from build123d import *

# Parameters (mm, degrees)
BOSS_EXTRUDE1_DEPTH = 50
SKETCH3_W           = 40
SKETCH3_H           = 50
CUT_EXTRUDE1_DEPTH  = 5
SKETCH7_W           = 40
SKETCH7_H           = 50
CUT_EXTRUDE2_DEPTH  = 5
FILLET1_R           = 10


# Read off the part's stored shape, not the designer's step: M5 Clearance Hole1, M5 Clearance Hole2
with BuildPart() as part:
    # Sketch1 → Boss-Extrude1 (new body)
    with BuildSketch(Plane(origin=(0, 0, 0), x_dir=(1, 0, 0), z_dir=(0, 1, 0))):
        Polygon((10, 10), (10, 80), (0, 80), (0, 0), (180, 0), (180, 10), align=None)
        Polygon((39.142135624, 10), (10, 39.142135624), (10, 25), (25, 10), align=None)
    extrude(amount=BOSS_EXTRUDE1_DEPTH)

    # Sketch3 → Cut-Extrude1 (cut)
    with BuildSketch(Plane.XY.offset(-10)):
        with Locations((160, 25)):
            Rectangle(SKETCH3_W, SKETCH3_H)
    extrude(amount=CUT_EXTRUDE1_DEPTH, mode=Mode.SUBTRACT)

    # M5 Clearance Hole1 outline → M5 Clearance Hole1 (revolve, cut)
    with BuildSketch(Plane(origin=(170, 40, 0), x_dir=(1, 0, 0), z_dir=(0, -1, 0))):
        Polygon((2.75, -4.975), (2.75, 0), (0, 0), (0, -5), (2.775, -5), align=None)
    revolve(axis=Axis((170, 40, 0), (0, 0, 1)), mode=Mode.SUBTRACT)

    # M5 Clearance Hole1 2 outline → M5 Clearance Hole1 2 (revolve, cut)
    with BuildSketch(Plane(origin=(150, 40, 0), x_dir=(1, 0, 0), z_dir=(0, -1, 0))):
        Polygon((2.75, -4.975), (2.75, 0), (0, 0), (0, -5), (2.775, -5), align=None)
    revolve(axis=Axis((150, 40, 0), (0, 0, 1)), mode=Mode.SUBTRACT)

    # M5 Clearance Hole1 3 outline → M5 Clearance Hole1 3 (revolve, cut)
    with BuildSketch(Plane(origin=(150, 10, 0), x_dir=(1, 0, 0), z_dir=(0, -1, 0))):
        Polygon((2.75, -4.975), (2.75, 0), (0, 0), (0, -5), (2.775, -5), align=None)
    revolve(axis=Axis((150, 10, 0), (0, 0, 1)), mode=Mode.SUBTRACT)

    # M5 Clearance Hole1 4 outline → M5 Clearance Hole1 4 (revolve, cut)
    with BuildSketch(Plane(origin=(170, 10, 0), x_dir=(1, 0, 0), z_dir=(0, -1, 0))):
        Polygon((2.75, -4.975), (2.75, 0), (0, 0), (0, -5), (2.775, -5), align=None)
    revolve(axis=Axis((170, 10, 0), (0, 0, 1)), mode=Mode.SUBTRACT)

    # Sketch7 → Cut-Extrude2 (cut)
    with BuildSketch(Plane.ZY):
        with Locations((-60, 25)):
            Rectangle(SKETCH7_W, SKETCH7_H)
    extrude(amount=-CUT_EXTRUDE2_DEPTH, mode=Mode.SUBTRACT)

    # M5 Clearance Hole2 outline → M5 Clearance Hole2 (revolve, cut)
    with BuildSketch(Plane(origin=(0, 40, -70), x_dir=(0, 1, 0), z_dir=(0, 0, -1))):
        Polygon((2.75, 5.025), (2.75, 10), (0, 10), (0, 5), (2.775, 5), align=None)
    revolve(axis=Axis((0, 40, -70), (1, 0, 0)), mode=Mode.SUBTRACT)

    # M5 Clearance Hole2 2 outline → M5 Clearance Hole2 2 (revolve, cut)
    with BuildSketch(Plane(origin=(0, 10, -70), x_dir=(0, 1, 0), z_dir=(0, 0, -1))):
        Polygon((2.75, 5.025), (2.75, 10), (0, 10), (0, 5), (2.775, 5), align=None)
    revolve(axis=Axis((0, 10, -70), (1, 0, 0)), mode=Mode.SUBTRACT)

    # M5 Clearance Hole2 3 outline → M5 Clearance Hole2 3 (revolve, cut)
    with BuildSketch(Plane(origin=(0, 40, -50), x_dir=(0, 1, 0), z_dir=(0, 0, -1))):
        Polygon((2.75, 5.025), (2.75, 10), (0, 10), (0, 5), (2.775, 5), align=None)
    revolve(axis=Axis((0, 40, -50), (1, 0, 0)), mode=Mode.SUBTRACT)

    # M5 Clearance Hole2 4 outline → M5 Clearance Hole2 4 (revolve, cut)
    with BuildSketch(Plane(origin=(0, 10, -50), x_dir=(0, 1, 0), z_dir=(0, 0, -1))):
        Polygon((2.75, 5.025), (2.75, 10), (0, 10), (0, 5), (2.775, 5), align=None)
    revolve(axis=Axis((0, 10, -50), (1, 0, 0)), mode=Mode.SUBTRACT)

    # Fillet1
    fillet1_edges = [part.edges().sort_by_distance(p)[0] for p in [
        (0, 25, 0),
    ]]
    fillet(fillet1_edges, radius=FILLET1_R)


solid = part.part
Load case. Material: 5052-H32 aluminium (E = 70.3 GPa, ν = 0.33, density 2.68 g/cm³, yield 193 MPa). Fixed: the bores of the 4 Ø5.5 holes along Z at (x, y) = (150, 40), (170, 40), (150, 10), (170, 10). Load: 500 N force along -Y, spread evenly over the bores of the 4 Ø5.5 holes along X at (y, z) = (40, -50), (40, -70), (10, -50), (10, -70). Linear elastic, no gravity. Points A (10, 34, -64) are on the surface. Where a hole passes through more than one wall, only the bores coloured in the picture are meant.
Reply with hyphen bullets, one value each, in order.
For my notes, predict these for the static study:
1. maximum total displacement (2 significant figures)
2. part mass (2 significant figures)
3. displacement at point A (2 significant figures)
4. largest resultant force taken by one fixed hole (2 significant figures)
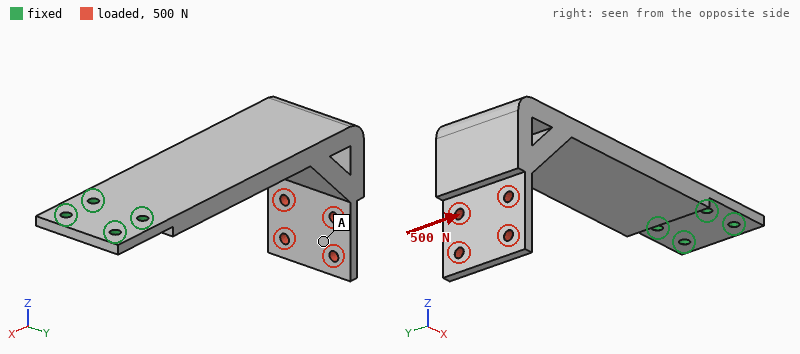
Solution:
- 0.69 mm
- 320 g
- 0.54 mm
- 2.1 kN
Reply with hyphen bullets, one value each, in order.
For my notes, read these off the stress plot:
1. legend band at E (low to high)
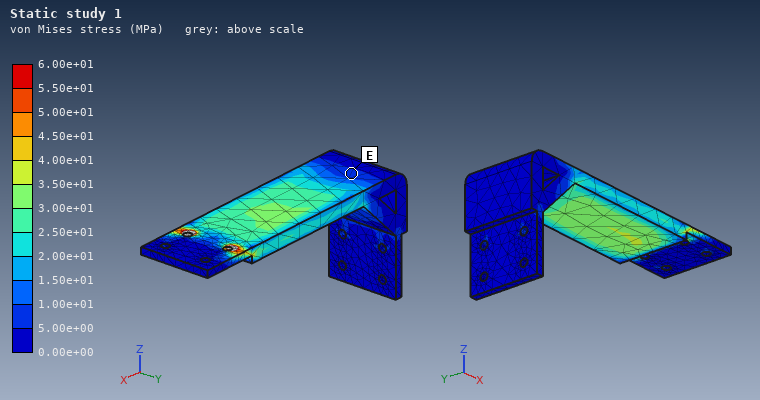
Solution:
- 5.00e+00 to 1.00e+01 MPa
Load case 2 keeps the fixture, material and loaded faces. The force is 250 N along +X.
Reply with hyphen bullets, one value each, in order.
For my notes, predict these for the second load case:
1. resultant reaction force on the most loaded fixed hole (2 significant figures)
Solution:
- 140 N
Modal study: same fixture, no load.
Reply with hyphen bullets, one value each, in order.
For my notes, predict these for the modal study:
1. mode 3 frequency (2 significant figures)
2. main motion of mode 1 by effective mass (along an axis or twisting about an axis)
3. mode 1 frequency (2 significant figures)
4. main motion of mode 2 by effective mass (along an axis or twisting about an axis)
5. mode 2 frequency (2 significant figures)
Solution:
- 1100 Hz
- along Z
- 130 Hz
- along Y
- 680 Hz
